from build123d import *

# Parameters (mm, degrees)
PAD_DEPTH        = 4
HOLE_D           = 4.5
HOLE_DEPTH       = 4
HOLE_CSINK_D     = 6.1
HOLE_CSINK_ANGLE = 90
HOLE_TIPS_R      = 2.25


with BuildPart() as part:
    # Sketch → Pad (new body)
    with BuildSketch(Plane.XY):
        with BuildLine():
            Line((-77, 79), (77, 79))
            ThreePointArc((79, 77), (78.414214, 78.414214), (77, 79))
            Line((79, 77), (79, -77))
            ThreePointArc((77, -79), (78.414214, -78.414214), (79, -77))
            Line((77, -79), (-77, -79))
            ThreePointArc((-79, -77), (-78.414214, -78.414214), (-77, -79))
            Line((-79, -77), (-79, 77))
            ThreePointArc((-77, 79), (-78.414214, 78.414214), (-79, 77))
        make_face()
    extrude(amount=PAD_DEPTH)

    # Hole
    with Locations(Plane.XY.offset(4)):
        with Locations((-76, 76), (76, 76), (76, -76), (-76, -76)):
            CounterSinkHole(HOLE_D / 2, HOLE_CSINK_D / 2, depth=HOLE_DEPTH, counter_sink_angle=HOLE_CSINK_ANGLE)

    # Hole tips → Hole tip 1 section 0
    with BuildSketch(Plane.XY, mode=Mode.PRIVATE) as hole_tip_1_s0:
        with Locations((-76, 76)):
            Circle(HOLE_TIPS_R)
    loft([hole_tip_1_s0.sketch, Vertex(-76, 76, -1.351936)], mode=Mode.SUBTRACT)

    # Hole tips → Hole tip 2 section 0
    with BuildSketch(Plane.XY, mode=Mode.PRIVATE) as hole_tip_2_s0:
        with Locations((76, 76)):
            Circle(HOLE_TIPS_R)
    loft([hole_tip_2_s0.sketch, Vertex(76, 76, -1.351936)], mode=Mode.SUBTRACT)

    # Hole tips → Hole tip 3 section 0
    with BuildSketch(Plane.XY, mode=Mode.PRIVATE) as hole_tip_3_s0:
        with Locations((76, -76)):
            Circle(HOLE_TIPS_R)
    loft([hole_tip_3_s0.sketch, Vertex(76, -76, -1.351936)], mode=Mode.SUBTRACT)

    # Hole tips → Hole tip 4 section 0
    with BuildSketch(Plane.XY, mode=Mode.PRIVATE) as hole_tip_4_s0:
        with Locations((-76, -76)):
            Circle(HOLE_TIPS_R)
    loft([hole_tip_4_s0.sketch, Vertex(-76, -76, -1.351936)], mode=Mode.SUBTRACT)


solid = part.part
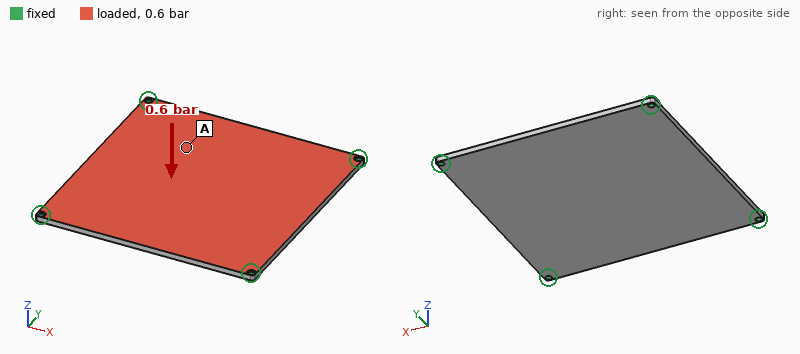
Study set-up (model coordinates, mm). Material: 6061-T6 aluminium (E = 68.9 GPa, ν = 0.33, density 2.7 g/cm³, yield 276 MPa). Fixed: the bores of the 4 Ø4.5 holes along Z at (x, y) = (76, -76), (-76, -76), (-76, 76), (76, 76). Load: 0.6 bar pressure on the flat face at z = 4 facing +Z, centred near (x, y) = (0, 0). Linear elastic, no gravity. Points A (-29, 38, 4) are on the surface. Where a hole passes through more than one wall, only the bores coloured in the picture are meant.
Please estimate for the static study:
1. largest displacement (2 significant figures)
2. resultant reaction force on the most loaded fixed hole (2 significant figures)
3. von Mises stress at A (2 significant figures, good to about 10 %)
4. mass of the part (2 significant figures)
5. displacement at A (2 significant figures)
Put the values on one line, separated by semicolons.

0.86 mm; 400 N; 29 MPa; 270 g; 0.66 mm
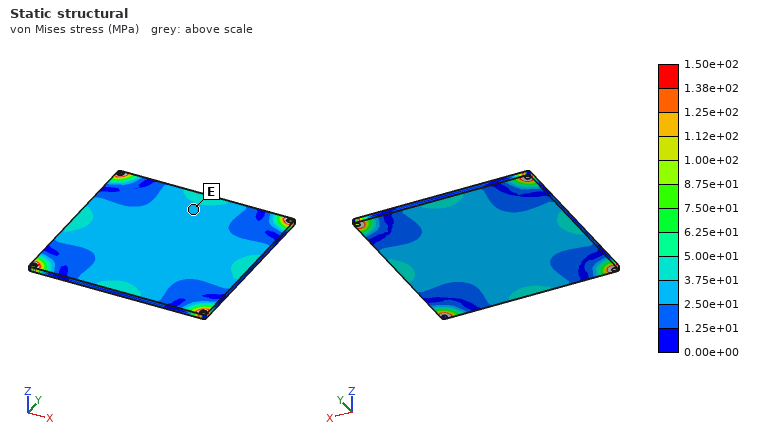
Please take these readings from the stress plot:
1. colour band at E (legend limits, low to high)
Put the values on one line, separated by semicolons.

2.50e+01 to 3.75e+01 MPa
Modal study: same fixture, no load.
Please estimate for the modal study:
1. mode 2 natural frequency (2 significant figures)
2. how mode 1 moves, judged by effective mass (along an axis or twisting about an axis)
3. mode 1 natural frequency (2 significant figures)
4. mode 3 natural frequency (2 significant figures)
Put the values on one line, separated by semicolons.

910 Hz; along Z; 480 Hz; 910 Hz
